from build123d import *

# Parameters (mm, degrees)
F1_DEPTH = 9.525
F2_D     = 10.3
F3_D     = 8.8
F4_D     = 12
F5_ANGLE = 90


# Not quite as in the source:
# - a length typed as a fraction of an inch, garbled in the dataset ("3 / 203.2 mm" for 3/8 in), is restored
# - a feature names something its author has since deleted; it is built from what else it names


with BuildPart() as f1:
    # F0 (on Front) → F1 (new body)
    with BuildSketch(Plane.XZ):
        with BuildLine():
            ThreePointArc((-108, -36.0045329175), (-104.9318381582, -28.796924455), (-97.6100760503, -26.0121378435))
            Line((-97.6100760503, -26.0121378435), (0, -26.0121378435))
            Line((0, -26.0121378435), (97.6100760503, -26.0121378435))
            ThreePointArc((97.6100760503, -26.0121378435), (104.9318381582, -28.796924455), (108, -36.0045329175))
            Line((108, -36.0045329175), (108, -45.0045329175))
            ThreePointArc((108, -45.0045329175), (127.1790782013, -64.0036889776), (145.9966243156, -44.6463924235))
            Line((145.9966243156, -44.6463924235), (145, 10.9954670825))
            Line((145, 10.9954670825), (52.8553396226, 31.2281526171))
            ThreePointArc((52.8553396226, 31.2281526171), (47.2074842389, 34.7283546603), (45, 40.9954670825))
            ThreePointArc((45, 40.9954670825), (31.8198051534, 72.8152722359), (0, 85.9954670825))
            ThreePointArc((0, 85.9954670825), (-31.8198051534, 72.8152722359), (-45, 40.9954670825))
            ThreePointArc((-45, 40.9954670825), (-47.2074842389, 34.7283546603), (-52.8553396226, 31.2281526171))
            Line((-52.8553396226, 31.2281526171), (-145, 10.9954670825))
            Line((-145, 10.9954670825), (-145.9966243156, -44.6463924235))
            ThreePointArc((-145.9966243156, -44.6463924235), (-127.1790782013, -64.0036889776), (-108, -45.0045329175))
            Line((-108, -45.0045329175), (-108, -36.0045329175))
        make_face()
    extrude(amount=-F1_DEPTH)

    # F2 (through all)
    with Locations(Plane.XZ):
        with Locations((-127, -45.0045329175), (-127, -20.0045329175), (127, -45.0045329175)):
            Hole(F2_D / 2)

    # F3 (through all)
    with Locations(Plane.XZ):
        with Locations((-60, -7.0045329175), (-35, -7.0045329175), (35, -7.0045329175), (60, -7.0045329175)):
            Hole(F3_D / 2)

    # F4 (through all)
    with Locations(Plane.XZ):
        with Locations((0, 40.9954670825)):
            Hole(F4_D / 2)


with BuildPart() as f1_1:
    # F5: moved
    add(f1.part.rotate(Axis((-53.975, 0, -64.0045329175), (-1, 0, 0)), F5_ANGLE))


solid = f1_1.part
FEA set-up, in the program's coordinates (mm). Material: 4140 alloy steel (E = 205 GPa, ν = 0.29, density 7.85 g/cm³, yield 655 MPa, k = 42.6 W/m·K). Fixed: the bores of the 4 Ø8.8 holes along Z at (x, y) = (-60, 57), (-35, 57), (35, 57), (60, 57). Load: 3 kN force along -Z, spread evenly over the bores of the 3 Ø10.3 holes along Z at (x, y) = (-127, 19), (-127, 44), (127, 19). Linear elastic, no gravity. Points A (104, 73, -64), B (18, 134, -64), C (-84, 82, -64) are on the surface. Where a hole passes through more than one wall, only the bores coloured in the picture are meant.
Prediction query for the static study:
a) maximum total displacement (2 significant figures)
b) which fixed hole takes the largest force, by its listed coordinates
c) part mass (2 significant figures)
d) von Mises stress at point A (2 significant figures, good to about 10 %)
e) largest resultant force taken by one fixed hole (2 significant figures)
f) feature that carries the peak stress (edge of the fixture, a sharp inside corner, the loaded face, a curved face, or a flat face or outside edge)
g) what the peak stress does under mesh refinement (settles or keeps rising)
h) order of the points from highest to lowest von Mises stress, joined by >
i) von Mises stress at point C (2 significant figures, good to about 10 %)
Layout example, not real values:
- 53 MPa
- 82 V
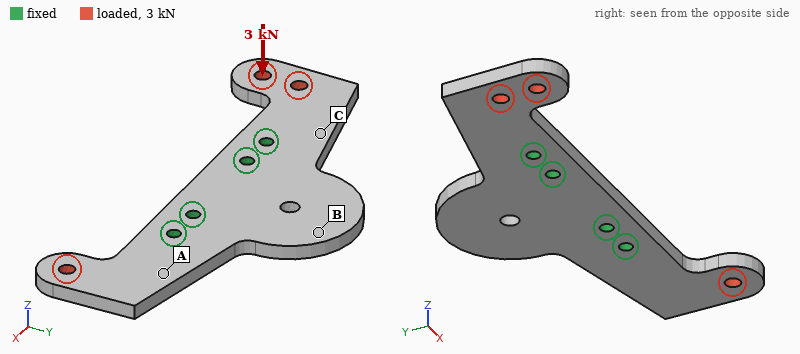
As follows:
- 0.57 mm
- (-60, 57)
- 1.6 kg
- 54 MPa
- 3.8 kN
- edge of the fixture
- keeps rising
- C > A > B
- 110 MPa
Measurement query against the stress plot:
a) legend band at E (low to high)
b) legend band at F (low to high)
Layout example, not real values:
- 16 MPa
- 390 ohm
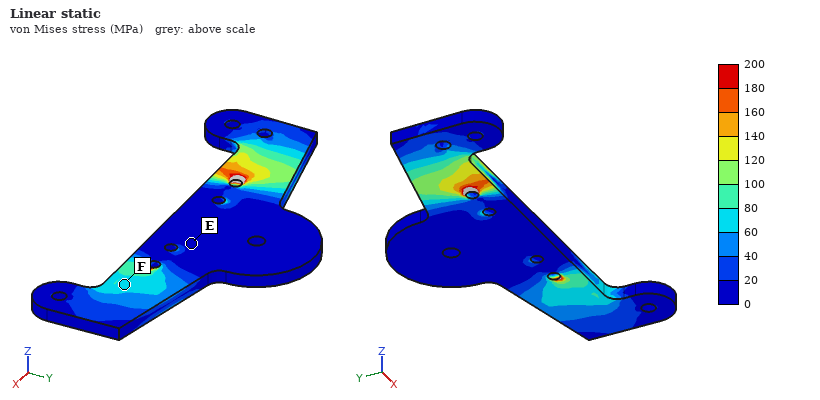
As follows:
- 0 to 20 MPa
- 60 to 80 MPa
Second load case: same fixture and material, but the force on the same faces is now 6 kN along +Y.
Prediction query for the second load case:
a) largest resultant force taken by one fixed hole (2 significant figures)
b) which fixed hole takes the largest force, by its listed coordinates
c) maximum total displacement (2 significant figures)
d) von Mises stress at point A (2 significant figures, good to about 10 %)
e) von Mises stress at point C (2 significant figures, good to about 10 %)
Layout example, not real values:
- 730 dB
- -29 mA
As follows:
- 7.6 kN
- (-60, 57)
- 63 µm
- 11 MPa
- 35 MPa
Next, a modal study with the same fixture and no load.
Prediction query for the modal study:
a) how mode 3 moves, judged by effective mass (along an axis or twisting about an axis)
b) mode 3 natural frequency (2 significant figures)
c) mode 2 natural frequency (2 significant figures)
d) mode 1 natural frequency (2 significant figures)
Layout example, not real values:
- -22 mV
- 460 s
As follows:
- along Z
- 1200 Hz
- 850 Hz
- 840 Hz
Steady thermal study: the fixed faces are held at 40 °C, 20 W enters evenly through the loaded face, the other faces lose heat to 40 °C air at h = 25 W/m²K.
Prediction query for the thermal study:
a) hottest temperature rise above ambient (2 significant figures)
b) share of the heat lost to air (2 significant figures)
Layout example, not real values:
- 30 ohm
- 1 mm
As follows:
- 39 K
- 51 %
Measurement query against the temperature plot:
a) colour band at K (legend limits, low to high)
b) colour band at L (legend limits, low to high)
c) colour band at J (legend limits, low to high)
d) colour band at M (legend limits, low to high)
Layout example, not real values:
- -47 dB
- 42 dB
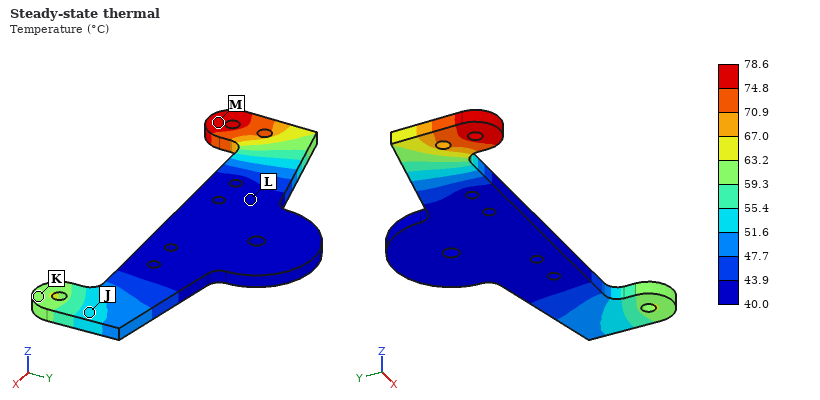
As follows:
- 59.3 to 63.2 °C
- 40.0 to 43.9 °C
- 51.6 to 55.4 °C
- 74.8 to 78.6 °C
